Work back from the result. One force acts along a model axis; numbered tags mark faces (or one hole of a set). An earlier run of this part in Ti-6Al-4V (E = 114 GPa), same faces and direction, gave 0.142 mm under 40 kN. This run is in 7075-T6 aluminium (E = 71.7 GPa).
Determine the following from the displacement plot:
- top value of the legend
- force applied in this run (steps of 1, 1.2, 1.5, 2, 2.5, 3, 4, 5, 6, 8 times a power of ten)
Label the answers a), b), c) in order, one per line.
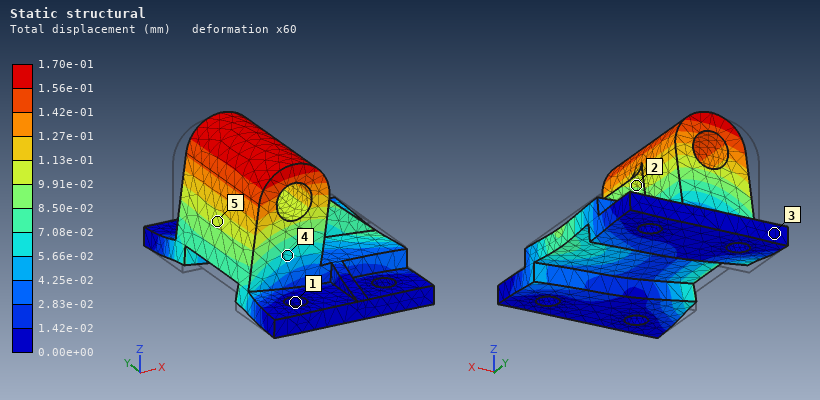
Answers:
a) 1.70e-01 mm
b) 30 kN
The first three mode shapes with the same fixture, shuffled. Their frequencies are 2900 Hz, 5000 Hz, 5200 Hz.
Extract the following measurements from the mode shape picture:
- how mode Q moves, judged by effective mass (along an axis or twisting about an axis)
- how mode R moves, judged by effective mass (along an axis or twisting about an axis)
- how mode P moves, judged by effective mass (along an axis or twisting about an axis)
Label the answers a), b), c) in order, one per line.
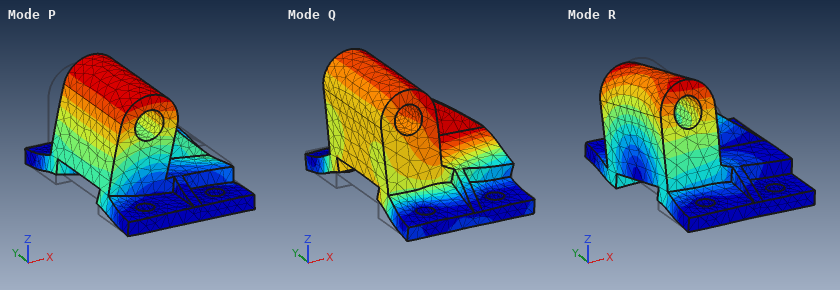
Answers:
a) along Z
b) along Y
c) along X
